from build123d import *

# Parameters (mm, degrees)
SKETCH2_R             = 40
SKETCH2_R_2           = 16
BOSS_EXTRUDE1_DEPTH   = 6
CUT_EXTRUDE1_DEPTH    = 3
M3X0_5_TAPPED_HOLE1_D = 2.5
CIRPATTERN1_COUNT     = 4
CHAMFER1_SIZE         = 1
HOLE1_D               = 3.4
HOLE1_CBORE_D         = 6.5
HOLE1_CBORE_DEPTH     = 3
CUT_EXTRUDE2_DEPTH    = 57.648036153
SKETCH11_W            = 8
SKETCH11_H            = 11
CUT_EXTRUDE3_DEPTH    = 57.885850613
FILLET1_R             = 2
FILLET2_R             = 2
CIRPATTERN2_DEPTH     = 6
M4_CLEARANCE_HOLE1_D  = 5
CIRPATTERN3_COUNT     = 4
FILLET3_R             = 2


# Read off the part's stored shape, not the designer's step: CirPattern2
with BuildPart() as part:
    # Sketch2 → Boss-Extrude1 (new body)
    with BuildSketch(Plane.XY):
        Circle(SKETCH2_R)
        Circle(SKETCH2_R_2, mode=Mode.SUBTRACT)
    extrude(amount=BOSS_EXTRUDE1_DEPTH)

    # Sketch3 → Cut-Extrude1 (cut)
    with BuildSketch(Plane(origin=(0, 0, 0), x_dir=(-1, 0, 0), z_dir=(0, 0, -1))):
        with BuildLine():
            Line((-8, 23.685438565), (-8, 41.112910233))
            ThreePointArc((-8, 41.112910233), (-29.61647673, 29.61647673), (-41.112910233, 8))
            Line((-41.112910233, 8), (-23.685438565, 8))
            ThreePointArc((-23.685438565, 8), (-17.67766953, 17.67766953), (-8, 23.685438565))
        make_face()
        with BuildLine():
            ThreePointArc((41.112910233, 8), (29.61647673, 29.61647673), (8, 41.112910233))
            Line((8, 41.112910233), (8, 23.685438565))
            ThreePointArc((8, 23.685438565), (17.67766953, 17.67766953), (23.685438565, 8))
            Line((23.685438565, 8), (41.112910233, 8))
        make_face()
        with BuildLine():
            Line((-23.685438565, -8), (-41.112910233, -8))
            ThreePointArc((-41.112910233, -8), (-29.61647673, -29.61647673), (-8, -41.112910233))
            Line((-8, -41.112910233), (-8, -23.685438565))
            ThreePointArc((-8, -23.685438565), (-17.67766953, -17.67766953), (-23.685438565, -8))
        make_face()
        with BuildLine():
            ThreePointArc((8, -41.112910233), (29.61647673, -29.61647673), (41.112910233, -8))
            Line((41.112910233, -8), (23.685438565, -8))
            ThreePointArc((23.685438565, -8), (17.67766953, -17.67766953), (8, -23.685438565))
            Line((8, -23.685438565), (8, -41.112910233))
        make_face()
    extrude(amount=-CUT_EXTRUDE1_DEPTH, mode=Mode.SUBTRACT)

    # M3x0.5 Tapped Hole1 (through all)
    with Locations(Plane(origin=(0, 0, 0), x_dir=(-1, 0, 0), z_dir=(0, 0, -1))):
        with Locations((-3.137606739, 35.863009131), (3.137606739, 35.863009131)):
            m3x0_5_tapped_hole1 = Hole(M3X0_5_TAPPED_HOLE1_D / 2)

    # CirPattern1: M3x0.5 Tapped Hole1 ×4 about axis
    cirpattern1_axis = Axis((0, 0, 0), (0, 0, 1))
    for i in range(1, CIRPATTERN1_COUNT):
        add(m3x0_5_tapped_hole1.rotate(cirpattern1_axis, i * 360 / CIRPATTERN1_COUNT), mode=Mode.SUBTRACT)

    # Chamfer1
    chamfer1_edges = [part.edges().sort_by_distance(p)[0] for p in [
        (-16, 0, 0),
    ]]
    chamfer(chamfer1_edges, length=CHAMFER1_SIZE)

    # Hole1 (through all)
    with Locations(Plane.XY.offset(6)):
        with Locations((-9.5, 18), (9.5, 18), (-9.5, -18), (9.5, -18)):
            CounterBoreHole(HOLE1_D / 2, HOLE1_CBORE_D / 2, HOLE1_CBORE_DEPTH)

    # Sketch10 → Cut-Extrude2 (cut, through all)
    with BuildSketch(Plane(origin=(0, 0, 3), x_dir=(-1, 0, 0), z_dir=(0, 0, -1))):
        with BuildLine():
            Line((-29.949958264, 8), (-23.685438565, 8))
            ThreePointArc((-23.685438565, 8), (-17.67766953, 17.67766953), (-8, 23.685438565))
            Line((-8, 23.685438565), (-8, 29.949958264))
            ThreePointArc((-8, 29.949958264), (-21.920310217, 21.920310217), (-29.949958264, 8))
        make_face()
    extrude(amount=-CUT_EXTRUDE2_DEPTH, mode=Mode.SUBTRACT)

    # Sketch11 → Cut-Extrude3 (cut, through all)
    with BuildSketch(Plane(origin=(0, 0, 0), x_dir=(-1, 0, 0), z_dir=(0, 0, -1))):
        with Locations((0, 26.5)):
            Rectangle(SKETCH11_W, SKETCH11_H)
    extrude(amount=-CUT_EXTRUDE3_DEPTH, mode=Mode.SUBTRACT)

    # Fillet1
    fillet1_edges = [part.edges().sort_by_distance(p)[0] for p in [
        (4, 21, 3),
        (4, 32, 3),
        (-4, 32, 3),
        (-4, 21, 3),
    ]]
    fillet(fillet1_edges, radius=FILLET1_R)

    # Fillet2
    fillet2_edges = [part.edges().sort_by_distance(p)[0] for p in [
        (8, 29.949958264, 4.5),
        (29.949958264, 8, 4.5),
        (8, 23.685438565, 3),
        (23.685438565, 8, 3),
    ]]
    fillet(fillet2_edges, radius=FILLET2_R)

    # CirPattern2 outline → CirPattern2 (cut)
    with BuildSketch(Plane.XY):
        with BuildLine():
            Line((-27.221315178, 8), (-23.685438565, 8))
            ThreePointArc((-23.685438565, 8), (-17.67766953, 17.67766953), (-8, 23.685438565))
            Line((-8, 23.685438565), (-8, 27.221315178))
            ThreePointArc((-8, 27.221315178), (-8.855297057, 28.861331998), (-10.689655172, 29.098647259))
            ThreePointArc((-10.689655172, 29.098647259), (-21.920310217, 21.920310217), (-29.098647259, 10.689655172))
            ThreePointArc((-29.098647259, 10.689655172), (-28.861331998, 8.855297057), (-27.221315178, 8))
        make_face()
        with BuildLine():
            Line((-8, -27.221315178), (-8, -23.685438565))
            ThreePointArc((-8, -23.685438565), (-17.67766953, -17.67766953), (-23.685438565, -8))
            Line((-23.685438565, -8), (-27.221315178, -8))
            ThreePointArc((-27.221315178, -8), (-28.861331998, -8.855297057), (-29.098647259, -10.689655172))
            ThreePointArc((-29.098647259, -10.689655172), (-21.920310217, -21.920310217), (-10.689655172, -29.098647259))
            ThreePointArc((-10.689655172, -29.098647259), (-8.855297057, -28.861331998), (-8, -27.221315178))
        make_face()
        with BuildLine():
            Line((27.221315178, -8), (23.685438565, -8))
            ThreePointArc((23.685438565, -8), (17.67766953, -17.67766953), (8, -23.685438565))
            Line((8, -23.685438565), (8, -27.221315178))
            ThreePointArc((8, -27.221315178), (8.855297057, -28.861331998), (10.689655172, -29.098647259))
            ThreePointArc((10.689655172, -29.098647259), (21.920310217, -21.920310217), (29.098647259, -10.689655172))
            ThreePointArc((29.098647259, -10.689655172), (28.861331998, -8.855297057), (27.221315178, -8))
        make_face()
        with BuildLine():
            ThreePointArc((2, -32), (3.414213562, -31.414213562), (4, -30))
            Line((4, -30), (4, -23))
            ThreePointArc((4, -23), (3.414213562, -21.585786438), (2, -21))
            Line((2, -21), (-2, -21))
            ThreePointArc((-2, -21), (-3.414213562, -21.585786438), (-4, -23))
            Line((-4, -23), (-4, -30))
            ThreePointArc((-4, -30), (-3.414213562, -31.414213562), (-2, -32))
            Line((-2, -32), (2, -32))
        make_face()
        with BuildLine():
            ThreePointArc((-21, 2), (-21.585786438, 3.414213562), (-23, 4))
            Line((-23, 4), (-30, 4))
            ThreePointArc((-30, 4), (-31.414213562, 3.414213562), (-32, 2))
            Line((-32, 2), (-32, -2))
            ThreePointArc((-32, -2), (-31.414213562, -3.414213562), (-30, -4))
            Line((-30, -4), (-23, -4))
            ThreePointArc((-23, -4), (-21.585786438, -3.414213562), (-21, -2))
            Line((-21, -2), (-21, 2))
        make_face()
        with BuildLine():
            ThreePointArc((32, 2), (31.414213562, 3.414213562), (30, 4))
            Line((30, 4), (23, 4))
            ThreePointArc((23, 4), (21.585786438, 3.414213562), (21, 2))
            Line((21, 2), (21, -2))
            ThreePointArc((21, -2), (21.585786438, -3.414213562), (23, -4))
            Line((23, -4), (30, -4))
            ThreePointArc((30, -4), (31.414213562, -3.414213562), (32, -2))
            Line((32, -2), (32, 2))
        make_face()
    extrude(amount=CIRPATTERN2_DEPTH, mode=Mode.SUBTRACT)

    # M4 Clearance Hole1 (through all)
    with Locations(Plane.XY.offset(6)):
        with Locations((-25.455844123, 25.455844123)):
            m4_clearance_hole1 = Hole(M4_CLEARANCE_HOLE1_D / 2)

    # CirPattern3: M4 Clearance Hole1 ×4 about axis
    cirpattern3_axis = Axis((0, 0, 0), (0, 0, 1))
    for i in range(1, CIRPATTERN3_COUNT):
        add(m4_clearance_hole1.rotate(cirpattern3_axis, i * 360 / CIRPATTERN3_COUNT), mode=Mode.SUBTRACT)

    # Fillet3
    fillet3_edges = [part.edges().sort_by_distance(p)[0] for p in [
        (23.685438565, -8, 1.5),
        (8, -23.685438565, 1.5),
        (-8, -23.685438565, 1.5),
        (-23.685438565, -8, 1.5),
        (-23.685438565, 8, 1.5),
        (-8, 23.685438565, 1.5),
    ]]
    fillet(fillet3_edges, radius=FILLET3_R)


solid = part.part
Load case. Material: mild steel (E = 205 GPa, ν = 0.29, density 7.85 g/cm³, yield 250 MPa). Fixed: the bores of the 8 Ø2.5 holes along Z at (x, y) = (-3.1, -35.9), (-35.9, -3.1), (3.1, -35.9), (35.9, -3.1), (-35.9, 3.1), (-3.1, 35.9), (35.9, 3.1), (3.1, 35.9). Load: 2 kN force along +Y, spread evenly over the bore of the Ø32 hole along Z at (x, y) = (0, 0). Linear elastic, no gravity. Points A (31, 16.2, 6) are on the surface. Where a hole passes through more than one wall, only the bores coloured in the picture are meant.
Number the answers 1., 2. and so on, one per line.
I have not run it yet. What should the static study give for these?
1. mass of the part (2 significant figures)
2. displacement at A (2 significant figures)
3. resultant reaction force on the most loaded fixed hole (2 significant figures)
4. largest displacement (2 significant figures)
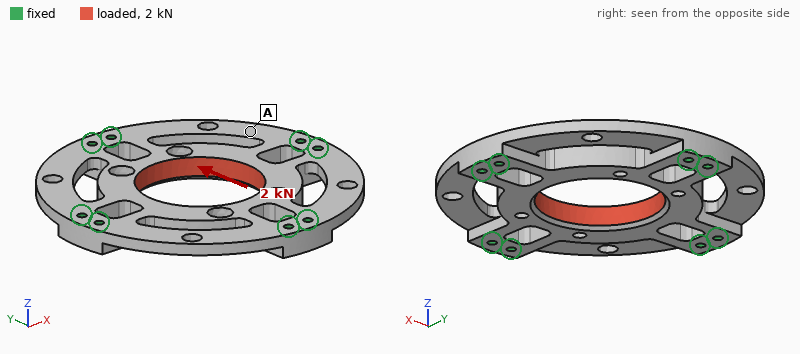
1. 110 g
2. 0.75 µm
3. 370 N
4. 3.5 µm
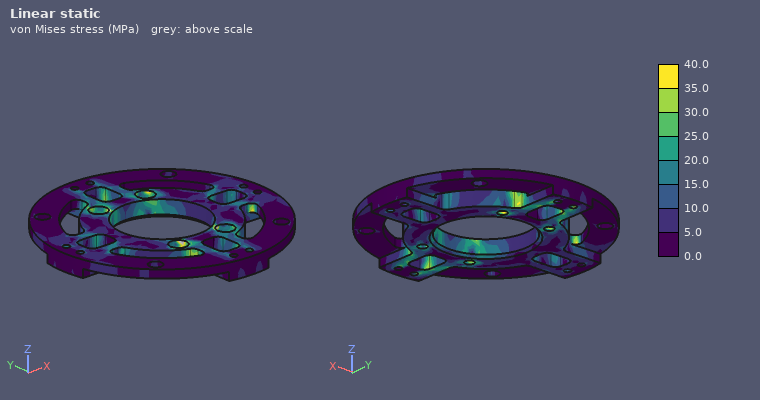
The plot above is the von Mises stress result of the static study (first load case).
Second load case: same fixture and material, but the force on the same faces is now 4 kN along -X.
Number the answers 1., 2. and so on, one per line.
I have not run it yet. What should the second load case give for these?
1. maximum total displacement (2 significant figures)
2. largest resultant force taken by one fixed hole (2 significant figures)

1. 5.2 µm
2. 780 N
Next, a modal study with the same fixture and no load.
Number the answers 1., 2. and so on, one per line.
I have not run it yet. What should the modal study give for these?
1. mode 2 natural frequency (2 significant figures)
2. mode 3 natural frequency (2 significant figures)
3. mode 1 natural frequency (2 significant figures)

1. 8000 Hz
2. 8000 Hz
3. 8000 Hz
